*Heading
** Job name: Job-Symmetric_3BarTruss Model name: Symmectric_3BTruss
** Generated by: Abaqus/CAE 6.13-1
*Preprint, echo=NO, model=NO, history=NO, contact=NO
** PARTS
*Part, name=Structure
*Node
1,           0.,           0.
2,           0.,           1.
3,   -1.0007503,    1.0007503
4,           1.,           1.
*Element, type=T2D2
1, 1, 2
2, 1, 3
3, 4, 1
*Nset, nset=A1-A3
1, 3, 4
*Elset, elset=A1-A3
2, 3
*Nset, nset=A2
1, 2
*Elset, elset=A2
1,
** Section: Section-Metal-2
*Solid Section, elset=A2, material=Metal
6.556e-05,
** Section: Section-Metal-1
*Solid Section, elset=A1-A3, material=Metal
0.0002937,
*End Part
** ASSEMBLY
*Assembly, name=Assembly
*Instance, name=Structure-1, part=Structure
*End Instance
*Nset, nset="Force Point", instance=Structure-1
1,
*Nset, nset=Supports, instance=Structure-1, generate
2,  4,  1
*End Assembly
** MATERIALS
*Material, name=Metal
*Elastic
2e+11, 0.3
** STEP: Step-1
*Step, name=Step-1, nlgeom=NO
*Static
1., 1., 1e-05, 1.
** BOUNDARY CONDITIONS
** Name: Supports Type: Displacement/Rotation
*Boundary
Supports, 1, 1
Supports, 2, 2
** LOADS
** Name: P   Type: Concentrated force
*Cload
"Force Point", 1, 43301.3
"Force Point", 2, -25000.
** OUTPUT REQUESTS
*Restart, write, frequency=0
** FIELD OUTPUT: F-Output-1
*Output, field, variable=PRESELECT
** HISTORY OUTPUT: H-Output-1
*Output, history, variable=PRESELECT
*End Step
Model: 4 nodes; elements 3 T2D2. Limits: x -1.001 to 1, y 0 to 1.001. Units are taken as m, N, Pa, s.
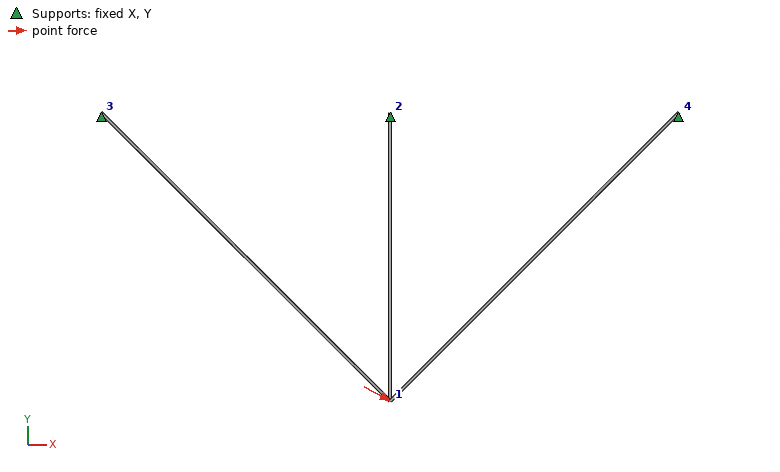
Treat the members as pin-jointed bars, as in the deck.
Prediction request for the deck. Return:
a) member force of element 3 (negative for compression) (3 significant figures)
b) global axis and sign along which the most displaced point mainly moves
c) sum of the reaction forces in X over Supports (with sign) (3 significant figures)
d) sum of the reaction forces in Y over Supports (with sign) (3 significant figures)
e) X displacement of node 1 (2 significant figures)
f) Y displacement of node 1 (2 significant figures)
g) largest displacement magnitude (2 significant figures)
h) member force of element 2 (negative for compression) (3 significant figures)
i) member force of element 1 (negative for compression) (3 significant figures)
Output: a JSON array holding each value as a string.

["-17200 N", "+X", "-43300 N", "25000 N", "0.0010 m", "-4.6e-04 m", "0.0011 m", "44100 N", "6000 N"]
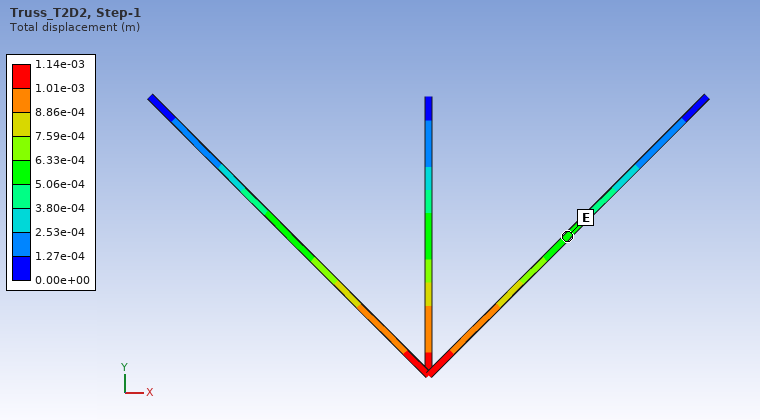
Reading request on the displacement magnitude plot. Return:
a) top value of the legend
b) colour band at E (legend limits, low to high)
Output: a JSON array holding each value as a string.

["1.14e-03 m", "5.06e-04 to 6.33e-04 m"]
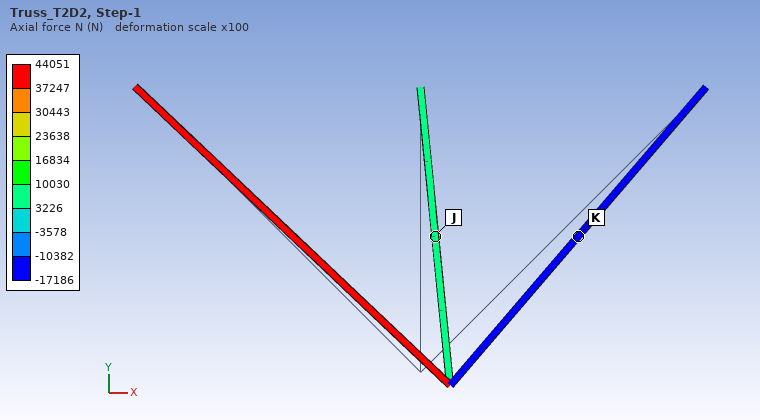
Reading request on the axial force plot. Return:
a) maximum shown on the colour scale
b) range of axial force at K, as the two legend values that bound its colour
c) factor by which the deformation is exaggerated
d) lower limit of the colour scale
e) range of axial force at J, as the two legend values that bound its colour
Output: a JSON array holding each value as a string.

["44051 N", "-17186 to -10382 N", "100", "-17186 N", "3226 to 10030 N"]
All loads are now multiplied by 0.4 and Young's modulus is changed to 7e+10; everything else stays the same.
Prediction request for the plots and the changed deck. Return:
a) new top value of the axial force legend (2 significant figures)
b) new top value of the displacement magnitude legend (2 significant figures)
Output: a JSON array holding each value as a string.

["18000 N", "0.0013 m"]
